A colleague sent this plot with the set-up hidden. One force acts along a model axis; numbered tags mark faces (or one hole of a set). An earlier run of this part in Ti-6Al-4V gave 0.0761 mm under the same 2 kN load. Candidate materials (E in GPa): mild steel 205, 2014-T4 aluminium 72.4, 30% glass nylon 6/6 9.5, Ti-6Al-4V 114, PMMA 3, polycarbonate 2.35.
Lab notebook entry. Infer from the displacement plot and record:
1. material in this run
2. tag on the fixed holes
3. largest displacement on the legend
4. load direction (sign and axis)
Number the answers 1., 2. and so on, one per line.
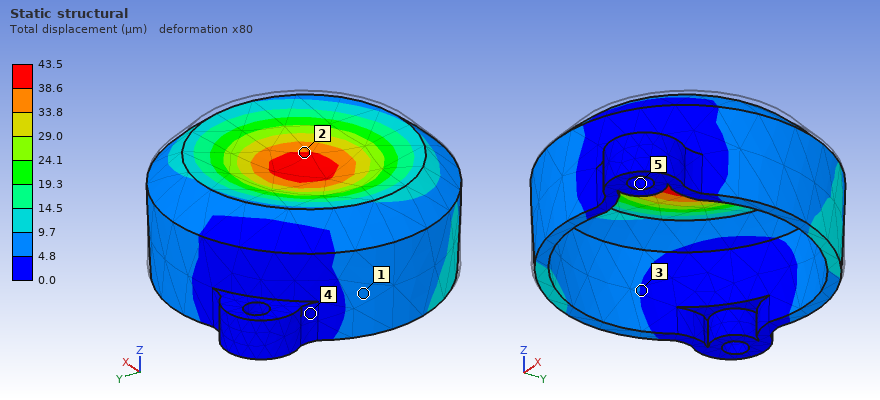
1. mild steel
2. 5
3. 43.5 µm
4. -Z
